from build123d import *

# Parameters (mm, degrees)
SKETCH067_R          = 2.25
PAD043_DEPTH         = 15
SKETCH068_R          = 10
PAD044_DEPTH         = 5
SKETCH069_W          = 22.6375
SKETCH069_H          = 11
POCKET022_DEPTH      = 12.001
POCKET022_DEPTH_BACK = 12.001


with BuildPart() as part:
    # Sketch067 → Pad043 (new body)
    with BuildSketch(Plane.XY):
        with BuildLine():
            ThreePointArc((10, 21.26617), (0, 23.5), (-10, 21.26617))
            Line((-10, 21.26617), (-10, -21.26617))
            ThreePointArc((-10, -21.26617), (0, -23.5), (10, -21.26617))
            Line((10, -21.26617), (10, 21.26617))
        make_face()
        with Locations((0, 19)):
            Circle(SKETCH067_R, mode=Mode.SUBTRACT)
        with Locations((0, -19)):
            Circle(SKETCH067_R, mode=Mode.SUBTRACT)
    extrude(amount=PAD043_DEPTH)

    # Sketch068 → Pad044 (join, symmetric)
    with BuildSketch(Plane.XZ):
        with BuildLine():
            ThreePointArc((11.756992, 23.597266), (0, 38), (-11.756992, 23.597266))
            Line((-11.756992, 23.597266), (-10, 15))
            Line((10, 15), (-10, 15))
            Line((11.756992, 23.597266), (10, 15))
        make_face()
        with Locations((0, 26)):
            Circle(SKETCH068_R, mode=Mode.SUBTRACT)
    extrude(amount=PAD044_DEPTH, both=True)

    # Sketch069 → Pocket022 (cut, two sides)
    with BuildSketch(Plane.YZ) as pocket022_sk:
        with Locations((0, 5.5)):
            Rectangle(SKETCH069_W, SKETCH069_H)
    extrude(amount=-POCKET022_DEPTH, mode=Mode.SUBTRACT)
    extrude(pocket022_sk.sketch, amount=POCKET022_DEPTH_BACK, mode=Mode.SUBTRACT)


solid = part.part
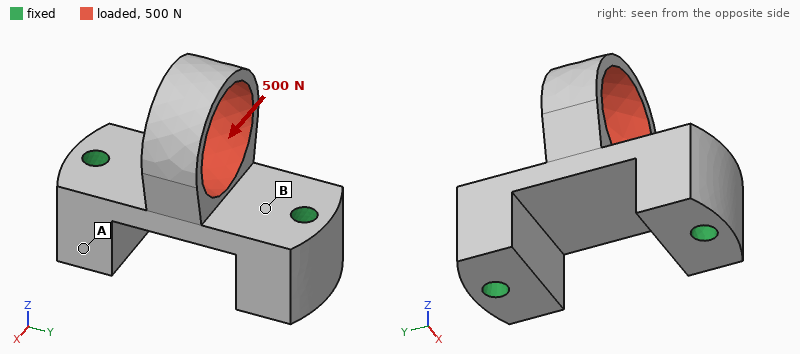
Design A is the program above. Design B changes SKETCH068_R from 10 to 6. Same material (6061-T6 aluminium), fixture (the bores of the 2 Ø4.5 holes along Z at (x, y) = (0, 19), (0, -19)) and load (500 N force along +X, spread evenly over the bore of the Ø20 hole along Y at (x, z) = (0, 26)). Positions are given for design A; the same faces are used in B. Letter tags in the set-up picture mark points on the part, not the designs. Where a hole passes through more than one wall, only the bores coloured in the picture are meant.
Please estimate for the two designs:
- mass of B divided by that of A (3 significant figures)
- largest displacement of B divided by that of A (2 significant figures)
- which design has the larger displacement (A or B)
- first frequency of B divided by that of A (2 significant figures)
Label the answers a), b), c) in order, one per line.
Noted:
a) 1.21
b) 0.32
c) A
d) 1.1
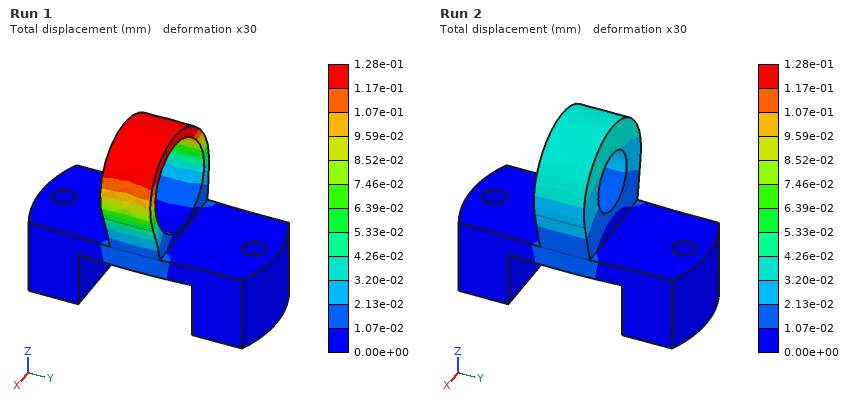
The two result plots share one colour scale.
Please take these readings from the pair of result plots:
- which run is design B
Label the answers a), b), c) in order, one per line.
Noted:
a) Run 2
